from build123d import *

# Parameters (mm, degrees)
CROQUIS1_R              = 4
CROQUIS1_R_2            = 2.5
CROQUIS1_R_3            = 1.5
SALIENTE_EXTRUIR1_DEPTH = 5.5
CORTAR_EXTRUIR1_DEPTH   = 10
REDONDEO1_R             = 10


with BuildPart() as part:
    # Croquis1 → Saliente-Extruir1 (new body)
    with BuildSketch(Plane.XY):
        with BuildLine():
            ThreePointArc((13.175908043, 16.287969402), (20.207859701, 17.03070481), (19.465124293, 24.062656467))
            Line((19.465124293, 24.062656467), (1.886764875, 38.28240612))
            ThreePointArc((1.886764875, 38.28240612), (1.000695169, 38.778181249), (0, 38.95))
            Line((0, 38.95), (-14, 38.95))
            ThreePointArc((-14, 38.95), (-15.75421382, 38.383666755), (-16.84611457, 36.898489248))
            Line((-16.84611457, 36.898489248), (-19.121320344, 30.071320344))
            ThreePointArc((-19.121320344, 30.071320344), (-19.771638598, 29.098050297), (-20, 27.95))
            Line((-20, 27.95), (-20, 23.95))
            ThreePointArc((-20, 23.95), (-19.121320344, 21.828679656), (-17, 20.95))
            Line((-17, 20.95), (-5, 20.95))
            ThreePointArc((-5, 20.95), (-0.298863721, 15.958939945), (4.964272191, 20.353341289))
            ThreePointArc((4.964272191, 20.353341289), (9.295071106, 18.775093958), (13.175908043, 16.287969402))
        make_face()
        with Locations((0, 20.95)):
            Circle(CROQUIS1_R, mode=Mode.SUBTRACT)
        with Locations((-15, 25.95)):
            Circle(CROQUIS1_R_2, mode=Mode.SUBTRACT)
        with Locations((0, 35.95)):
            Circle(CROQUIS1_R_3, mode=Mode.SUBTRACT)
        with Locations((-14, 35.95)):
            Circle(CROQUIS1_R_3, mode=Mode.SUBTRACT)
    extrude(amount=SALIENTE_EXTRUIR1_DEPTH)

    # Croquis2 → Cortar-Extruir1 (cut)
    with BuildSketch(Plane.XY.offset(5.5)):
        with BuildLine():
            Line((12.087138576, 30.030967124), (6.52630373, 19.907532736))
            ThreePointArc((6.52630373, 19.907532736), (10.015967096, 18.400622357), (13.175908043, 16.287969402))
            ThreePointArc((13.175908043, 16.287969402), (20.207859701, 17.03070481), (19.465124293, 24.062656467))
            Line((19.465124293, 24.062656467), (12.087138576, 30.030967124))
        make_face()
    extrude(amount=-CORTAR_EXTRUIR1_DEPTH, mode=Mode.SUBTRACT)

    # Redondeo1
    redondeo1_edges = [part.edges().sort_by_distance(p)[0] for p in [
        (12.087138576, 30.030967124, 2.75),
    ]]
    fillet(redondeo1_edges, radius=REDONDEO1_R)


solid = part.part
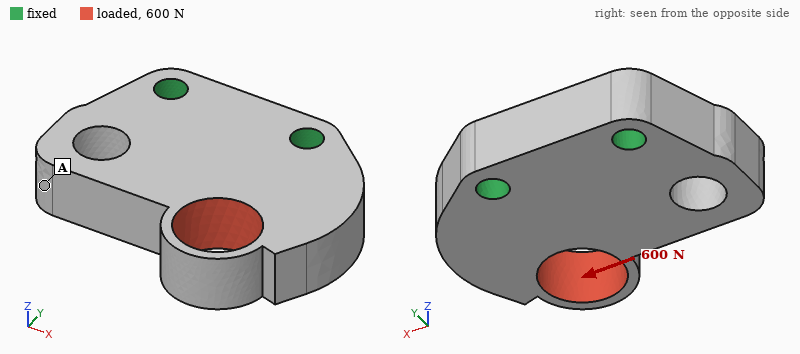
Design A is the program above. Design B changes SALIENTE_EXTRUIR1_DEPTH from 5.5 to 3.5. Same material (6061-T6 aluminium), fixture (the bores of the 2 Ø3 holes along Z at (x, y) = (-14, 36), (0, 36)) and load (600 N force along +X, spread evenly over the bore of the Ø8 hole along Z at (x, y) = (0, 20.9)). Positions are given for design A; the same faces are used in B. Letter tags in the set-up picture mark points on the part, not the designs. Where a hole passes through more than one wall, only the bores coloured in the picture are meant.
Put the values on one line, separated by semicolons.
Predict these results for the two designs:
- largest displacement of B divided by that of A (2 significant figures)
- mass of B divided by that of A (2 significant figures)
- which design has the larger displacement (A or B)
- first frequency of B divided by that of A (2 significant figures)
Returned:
1.6; 0.64; B; 0.71
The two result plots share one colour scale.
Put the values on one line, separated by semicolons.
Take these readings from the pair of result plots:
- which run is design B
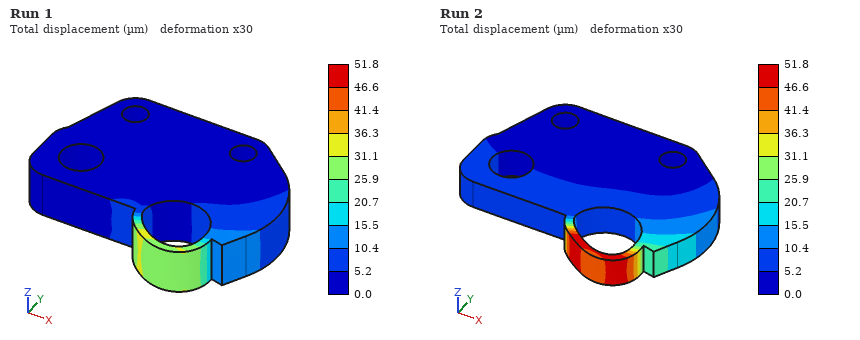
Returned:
Run 2
